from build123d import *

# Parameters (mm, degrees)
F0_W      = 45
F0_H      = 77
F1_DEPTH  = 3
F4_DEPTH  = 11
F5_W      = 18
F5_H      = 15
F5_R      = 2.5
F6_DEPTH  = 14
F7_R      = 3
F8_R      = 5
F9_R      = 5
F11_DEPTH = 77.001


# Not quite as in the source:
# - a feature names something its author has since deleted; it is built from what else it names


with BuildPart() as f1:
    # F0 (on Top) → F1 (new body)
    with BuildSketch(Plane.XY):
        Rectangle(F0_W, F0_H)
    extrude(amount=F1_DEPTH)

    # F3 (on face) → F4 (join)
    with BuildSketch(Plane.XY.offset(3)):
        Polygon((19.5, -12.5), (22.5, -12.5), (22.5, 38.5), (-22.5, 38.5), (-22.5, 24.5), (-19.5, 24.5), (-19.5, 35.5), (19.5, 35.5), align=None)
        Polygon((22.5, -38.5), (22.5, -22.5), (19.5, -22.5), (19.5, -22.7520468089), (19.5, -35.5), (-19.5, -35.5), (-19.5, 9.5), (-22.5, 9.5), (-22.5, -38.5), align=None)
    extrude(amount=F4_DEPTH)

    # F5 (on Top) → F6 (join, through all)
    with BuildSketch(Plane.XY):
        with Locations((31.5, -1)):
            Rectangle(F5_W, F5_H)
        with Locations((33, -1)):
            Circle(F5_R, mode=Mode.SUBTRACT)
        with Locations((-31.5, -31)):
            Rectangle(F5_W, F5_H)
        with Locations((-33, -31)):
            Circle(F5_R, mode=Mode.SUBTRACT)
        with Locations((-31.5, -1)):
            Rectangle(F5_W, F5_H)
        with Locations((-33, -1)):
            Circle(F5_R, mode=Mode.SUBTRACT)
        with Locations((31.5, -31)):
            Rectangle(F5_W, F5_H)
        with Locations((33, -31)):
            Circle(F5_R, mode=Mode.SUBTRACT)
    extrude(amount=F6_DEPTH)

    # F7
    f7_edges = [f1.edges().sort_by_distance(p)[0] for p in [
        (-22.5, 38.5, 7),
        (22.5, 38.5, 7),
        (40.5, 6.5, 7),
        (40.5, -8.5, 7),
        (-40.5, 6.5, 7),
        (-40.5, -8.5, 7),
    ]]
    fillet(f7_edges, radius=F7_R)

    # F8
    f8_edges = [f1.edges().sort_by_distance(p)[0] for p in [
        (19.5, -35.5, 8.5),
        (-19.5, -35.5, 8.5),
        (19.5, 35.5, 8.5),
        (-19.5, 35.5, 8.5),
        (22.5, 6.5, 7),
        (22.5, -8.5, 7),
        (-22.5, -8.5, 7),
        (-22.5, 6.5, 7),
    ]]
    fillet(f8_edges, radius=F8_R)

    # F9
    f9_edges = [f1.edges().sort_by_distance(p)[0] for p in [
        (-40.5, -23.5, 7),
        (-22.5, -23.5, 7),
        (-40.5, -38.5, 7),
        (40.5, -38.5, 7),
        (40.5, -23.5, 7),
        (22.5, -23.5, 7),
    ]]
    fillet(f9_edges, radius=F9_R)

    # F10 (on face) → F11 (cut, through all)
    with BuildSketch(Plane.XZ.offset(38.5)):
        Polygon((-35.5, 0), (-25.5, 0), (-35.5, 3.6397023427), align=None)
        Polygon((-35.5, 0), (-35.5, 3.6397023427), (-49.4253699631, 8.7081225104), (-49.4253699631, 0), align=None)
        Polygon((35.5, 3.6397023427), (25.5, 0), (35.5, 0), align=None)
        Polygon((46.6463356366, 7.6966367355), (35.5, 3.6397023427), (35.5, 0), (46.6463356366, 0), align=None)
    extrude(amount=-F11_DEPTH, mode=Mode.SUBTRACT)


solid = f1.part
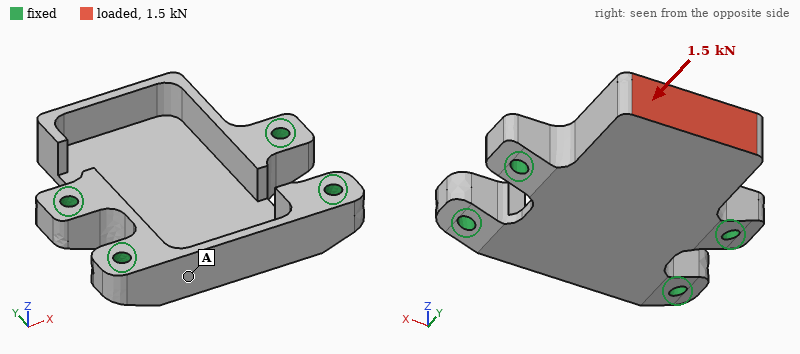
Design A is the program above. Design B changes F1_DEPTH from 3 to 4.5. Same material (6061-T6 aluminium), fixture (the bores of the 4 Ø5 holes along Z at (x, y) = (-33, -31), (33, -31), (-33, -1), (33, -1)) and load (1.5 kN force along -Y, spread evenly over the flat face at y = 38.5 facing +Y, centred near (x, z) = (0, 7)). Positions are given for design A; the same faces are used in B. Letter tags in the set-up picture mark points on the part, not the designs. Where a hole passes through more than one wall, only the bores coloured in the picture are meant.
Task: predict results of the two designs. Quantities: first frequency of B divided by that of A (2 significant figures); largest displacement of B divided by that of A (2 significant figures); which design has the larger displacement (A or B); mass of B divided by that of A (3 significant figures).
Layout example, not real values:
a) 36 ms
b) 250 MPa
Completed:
a) 1.3
b) 0.42
c) A
d) 1.14
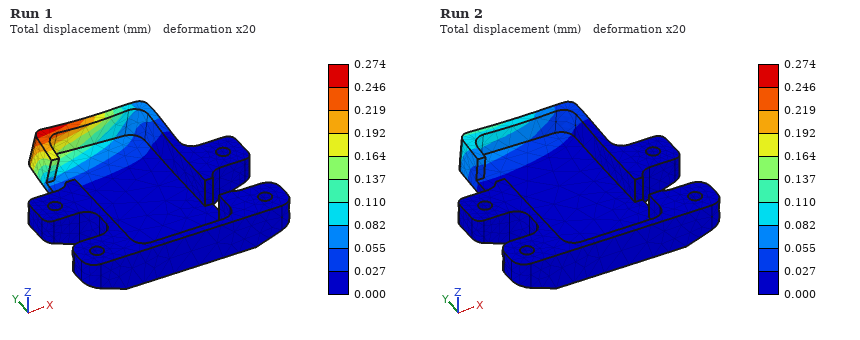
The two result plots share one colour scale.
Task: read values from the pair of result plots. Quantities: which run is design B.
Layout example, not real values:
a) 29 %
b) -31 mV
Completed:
a) Run 2
